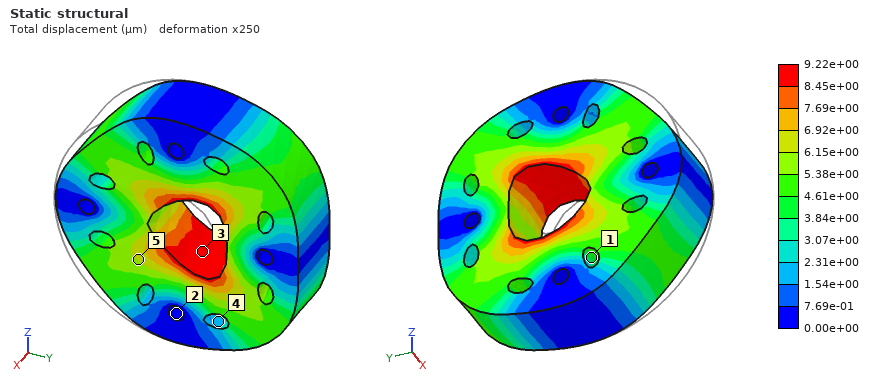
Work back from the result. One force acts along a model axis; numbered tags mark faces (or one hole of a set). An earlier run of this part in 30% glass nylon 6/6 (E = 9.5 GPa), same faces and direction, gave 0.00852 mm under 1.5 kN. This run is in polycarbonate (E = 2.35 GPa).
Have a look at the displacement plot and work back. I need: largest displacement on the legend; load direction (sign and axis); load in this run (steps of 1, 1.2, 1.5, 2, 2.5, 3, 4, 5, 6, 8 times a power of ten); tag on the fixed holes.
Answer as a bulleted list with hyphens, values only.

- 9.22e+00 µm
- +Y
- 400 N
- 2
